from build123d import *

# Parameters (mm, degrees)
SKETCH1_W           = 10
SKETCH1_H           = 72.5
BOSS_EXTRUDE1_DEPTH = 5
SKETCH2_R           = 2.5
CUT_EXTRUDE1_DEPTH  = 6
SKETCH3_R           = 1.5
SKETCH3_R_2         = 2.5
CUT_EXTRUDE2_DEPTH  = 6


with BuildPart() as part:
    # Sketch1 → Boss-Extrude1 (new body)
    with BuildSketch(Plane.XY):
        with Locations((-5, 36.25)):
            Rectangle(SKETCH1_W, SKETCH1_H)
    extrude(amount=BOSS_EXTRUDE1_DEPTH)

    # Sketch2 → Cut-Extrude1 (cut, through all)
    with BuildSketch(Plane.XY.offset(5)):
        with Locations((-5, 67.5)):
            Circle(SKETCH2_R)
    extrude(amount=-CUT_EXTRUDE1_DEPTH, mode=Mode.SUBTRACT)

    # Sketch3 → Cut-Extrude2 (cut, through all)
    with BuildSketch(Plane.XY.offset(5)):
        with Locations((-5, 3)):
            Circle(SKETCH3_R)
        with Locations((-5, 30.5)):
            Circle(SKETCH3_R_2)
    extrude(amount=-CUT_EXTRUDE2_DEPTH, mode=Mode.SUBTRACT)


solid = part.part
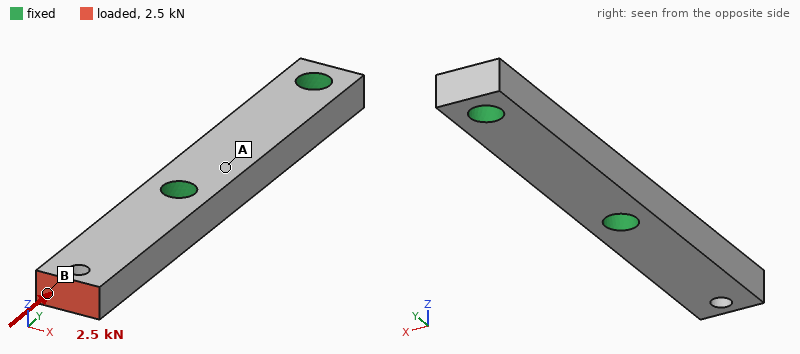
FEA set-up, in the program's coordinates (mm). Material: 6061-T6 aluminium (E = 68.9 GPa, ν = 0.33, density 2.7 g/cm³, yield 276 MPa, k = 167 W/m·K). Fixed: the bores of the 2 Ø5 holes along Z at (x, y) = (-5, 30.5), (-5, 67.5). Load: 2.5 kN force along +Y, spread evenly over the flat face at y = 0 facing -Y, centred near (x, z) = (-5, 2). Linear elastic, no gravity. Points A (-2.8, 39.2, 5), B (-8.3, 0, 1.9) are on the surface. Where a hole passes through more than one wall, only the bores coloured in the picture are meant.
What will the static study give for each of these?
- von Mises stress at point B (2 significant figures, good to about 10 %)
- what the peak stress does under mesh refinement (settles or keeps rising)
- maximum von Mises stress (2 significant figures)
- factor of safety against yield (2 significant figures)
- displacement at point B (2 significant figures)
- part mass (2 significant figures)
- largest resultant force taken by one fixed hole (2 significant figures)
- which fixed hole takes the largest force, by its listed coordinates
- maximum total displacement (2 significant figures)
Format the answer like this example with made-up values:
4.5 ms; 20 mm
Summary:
63 MPa; settles; 200 MPa; 1.4; 23 µm; 9.2 g; 2.5 kN; (-5, 30.5); 27 µm
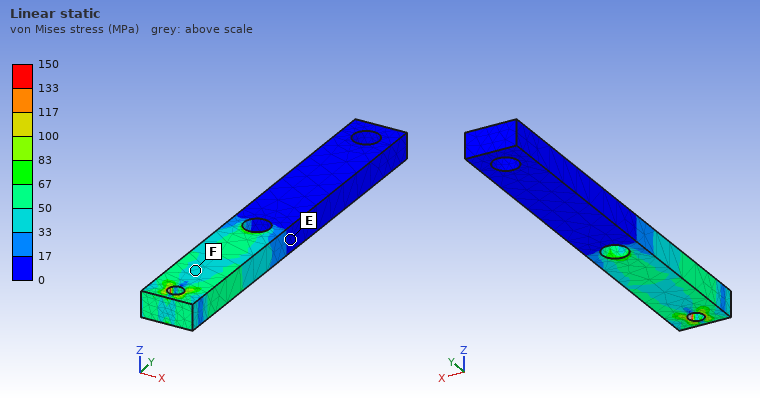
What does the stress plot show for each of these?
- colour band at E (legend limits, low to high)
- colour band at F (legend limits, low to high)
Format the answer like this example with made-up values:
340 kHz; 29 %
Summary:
0 to 17 MPa; 33 to 50 MPa
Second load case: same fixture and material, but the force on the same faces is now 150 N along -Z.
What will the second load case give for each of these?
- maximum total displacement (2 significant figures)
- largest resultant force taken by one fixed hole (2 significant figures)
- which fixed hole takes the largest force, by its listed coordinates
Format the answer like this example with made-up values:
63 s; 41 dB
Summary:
0.17 mm; 150 N; (-5, 30.5)
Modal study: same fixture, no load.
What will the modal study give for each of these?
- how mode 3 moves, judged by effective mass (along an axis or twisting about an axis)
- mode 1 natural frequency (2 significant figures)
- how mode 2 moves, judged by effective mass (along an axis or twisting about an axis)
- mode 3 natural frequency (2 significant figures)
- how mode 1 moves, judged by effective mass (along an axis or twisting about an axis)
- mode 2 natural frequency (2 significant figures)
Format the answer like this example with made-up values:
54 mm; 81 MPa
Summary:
along Z; 5000 Hz; along X; 20 kHz; along Z; 8200 Hz
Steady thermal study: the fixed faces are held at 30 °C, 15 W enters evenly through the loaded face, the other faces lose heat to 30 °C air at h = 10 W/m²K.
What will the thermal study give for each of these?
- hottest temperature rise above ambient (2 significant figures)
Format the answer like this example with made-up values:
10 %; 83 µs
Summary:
55 K
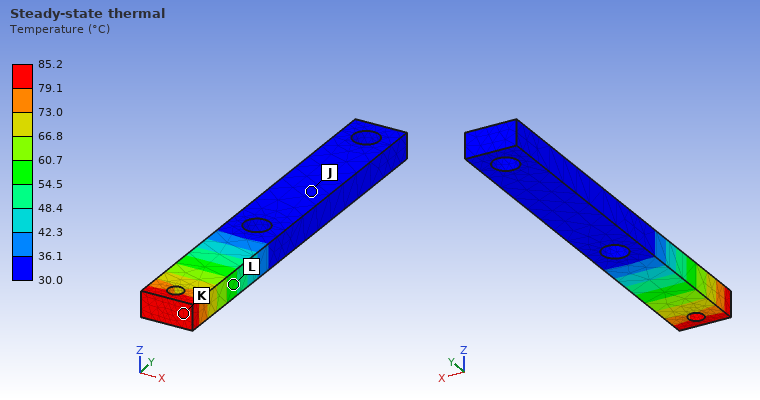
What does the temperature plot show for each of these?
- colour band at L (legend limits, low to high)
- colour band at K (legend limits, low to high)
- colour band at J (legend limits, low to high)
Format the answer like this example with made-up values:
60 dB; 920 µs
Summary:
54.5 to 60.7 °C; 79.1 to 85.2 °C; 30.0 to 36.1 °C
